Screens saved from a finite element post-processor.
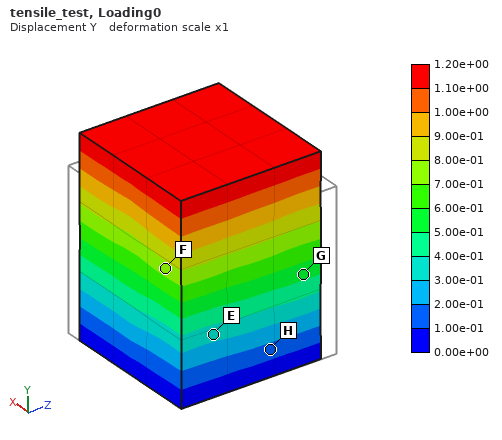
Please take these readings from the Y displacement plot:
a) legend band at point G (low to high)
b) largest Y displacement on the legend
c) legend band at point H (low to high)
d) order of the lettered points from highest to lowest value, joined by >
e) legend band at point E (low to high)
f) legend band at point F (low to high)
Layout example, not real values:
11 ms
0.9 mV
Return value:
5.00e-01 to 6.00e-01
1.20e+00
1.00e-01 to 2.00e-01
F > G > E > H
3.00e-01 to 4.00e-01
7.00e-01 to 8.00e-01
